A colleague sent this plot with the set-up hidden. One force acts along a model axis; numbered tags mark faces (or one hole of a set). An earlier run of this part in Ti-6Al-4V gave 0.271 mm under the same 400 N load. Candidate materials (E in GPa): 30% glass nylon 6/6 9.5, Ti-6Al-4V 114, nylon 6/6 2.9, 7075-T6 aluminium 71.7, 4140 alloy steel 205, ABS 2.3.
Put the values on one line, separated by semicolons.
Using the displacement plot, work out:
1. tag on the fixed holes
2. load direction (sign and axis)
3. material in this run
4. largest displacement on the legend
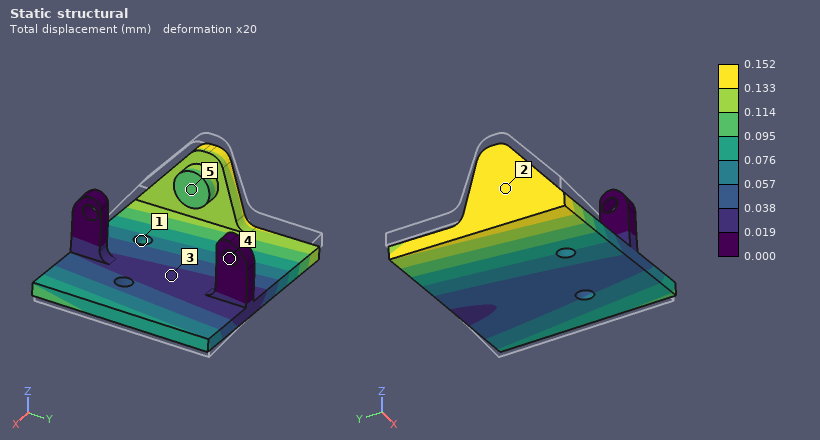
4; +X; 4140 alloy steel; 0.152 mm
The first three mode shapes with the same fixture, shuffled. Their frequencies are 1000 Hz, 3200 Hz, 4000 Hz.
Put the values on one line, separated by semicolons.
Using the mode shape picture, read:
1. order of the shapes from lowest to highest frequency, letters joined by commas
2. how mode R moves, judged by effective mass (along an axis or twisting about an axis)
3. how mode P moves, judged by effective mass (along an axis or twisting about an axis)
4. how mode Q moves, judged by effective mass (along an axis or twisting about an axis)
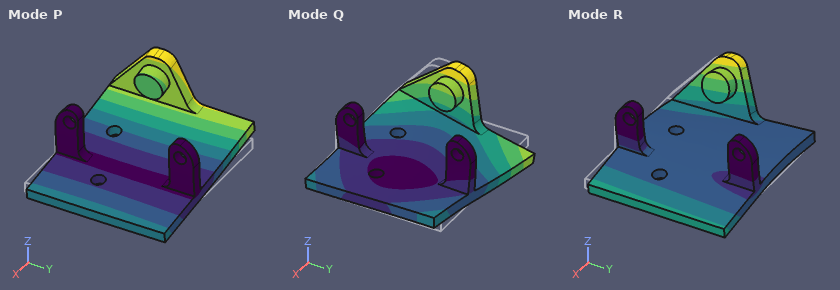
P, Q, R; along X; along Z; along Y
